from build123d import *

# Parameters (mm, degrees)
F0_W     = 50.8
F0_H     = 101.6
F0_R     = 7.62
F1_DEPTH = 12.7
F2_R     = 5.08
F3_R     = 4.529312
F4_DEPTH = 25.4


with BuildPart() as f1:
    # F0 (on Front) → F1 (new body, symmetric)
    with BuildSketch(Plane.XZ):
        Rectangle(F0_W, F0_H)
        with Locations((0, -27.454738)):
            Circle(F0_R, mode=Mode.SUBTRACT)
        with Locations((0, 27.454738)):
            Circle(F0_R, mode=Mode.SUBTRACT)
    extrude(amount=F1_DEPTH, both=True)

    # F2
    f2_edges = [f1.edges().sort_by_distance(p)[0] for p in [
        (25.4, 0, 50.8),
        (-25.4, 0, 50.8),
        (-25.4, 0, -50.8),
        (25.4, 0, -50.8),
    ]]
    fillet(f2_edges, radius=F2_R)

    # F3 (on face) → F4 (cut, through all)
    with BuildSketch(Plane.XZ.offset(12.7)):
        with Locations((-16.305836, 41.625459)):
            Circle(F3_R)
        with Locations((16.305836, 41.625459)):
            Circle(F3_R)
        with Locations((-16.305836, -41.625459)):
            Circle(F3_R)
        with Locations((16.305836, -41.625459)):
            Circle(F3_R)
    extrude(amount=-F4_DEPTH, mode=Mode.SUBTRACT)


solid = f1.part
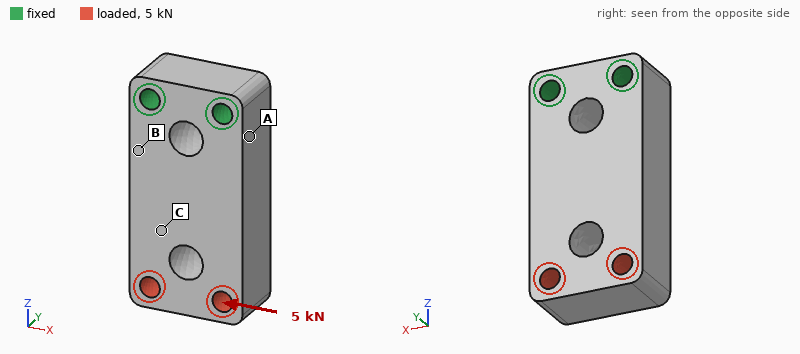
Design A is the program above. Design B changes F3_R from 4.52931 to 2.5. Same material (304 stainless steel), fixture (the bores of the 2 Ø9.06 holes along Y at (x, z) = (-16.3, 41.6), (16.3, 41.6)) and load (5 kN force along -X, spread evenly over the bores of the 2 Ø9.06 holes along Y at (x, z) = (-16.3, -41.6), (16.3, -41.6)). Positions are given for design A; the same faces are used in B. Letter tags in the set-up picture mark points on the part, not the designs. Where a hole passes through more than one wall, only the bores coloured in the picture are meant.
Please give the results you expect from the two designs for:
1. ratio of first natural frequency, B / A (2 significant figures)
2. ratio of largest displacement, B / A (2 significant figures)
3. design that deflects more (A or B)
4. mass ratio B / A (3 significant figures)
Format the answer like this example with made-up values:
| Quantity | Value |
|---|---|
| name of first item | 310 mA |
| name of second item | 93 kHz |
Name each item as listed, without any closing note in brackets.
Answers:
| Quantity | Value |
|---|---|
| ratio of first natural frequency, B / A | 0.90 |
| ratio of largest displacement, B / A | 1.1 |
| design that deflects more | B |
| mass ratio B / A | 1.04 |
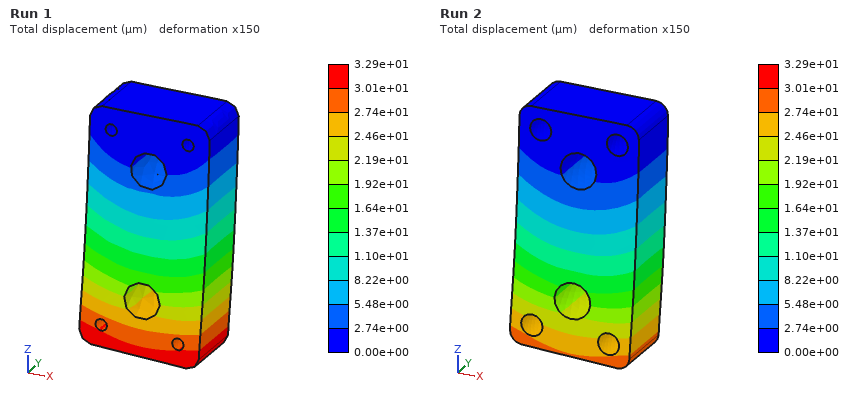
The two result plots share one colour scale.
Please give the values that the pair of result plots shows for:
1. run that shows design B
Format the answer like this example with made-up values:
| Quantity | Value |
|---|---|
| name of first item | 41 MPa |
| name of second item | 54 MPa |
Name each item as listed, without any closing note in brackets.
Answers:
| Quantity | Value |
|---|---|
| run that shows design B | Run 1 |
